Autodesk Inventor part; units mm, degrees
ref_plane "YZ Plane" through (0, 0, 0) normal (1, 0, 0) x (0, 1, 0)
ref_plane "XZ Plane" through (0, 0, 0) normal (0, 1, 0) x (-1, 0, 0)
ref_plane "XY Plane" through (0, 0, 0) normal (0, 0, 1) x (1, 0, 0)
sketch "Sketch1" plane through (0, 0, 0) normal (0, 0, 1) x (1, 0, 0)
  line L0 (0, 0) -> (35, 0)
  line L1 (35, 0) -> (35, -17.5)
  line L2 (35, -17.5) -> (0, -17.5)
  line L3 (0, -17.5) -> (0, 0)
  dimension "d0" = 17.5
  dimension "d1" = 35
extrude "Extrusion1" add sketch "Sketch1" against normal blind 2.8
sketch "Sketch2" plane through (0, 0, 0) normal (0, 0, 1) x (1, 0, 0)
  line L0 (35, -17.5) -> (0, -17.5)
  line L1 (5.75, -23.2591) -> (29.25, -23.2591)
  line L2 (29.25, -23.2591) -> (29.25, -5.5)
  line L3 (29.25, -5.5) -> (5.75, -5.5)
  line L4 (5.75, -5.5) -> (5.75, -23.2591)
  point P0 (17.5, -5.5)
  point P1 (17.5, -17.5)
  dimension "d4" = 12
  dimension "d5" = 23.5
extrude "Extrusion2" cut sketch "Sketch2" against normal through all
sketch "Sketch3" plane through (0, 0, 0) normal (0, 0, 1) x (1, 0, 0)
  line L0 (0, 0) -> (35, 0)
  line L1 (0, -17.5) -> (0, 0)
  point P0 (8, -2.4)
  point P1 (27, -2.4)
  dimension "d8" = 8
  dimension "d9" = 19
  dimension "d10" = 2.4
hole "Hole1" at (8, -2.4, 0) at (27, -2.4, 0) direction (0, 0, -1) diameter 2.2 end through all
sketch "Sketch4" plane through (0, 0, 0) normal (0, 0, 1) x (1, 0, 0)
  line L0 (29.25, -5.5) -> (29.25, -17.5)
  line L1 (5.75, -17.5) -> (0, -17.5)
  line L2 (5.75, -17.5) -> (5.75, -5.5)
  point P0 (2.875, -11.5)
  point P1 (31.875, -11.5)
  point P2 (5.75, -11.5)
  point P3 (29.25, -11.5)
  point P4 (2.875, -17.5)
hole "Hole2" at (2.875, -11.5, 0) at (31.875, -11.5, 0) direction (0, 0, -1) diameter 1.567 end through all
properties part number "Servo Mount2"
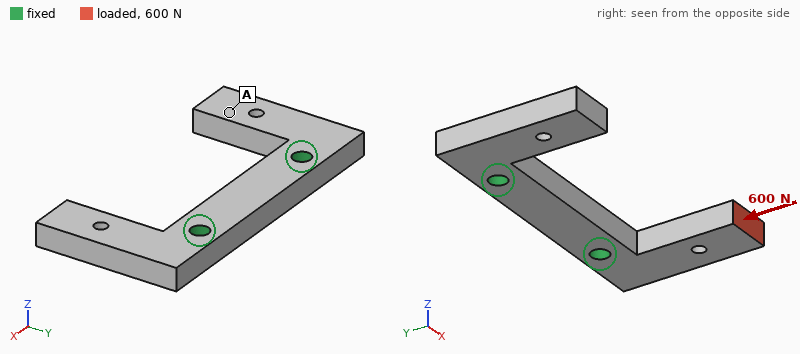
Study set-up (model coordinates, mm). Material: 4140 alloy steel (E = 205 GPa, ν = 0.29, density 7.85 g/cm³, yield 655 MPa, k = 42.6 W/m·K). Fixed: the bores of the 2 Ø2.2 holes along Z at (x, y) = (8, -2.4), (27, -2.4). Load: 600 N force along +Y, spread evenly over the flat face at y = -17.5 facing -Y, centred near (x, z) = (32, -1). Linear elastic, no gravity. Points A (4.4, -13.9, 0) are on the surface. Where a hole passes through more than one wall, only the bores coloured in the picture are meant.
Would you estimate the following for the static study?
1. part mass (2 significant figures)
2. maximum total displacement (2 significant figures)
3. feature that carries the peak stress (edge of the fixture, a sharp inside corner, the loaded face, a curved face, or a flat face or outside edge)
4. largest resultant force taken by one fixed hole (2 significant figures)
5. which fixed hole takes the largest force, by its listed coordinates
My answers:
7.0 g
28 µm
edge of the fixture
640 N
(27, -2.4)
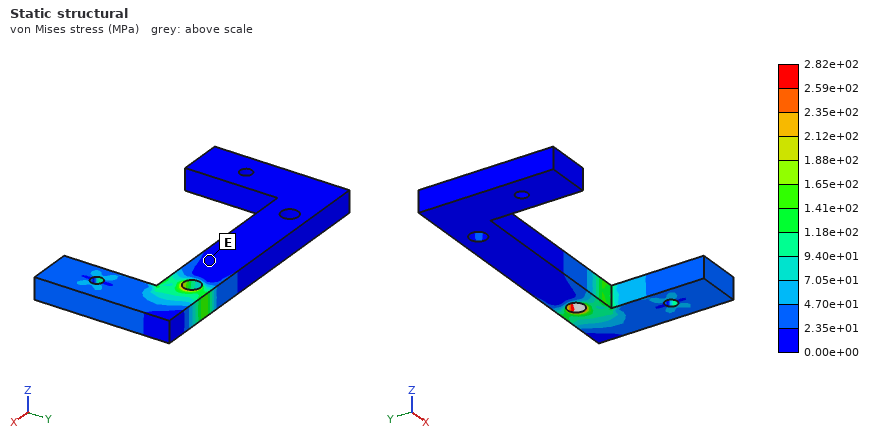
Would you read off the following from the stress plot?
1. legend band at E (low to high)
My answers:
0.00e+00 to 2.35e+01 MPa
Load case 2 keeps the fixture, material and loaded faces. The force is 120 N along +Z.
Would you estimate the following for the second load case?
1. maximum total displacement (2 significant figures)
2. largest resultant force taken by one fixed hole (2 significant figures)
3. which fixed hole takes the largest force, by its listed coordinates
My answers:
94 µm
120 N
(27, -2.4)
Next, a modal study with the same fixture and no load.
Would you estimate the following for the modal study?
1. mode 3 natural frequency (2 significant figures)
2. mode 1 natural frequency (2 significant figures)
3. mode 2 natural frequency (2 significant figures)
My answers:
13 kHz
8100 Hz
8100 Hz
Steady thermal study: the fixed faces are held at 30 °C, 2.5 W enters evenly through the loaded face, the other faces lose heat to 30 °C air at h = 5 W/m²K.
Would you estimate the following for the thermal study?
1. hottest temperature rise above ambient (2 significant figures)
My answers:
64 K
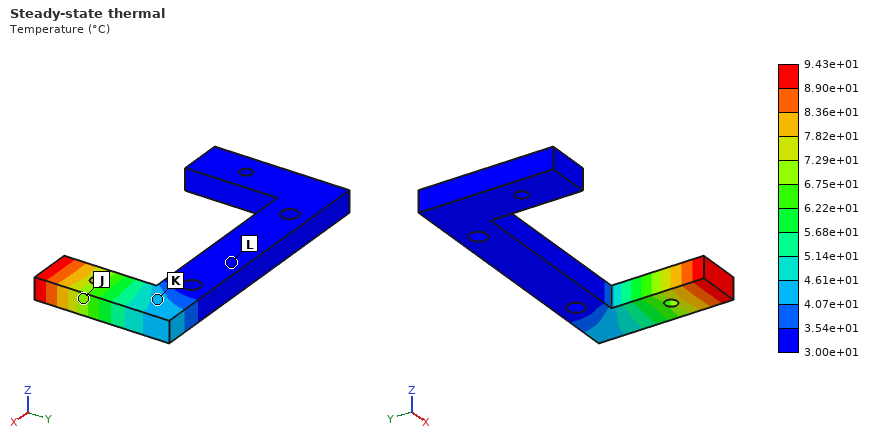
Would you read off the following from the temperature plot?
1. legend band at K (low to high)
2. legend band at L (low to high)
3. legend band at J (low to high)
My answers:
4.07e+01 to 4.61e+01 °C
3.00e+01 to 3.54e+01 °C
6.75e+01 to 7.29e+01 °C
